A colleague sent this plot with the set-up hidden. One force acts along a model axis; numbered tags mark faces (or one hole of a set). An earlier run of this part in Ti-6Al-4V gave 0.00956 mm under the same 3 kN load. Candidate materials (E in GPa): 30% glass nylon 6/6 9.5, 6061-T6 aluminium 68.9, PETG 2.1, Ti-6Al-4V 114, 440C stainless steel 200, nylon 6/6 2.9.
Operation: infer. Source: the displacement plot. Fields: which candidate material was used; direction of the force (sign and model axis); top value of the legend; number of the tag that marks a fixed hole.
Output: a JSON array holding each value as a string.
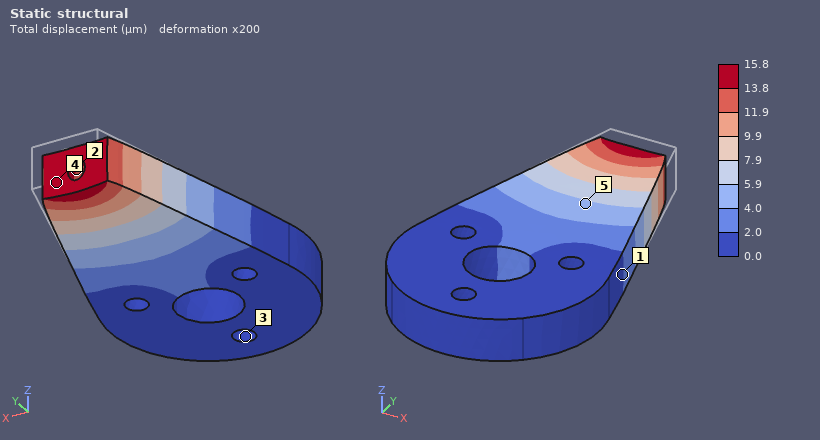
["6061-T6 aluminium", "-Y", "15.8 µm", "3"]
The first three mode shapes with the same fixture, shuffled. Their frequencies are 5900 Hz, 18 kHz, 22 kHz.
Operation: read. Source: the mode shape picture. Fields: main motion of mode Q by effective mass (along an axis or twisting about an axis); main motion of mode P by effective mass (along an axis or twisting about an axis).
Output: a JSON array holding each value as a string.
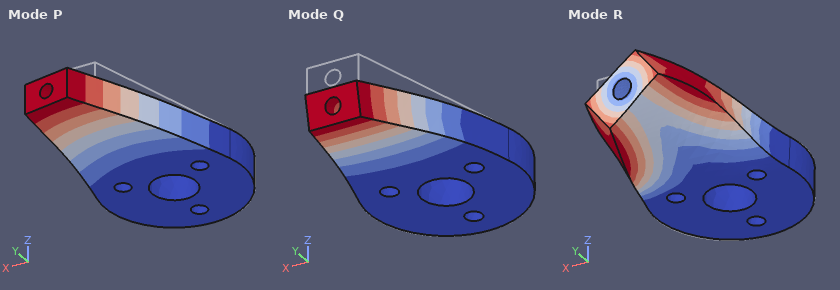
["along Z", "along X"]
